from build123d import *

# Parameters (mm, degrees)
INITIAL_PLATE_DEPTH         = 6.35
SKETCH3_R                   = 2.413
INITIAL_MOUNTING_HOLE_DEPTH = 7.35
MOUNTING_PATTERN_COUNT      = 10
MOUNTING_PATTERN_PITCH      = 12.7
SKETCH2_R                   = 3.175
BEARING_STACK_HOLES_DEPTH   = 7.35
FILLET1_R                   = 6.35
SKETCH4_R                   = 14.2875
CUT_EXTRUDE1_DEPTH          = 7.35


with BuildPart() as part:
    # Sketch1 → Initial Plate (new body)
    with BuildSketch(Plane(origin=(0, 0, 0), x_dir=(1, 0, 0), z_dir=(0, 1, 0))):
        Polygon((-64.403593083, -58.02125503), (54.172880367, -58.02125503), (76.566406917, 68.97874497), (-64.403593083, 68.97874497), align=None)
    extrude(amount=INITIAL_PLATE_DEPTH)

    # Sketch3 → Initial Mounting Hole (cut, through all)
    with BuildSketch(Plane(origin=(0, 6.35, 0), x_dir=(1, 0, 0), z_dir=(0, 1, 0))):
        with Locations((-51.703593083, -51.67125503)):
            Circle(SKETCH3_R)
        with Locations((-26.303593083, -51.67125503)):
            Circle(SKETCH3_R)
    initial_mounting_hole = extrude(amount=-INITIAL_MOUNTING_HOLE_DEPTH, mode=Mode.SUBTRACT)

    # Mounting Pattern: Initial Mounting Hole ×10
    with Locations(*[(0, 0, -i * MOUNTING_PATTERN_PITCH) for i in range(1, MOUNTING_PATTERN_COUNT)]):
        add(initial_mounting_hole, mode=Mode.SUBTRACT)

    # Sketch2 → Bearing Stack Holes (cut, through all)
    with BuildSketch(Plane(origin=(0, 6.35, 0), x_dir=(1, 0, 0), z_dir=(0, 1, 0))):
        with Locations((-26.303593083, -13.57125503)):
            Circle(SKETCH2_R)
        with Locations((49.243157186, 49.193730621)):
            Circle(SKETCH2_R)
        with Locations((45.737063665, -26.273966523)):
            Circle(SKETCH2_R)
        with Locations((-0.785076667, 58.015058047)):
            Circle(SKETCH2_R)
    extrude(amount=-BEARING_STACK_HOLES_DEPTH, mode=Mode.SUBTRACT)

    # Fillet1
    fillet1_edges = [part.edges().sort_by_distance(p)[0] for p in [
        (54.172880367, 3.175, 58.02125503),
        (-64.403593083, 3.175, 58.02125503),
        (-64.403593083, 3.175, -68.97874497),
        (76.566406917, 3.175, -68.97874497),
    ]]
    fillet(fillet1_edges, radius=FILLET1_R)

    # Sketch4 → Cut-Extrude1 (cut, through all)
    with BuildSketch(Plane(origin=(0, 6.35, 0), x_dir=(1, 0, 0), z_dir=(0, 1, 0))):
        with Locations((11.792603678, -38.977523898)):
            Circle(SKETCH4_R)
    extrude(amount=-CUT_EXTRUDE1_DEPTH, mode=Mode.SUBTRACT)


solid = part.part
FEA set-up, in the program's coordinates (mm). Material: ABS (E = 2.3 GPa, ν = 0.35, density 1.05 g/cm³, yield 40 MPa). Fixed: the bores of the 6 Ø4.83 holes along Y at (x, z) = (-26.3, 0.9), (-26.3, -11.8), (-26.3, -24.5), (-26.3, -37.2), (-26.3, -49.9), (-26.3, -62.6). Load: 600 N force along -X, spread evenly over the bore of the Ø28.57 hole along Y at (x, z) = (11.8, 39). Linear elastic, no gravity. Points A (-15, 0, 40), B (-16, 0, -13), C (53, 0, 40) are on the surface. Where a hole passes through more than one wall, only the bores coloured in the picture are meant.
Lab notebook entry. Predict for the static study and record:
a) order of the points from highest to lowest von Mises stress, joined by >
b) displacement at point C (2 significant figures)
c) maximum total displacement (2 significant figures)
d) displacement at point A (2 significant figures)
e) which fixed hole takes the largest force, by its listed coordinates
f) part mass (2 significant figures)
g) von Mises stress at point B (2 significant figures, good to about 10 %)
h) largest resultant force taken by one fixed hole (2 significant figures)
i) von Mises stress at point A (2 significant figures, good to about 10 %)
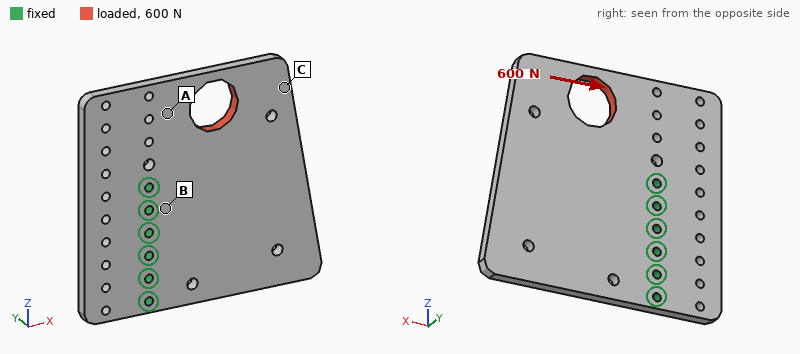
B > A > C
0.23 mm
0.27 mm
0.15 mm
(-26.3, 0.9)
100 g
2.3 MPa
760 N
1.5 MPa
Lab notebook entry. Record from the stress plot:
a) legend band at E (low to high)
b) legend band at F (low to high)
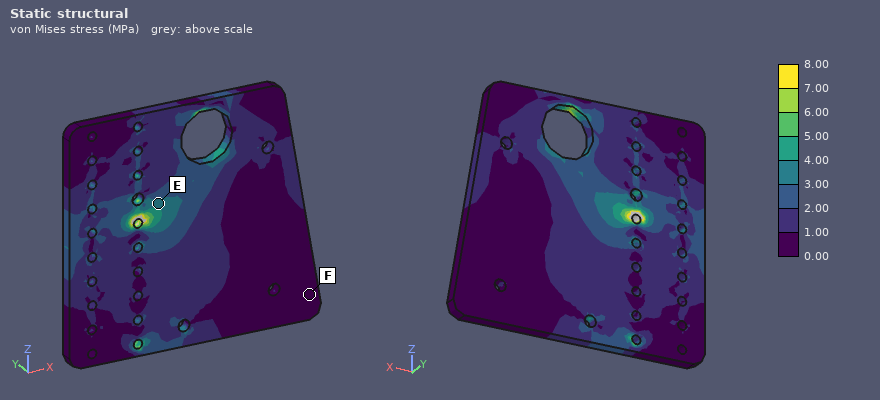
3.00 to 4.00 MPa
0.00 to 1.00 MPa
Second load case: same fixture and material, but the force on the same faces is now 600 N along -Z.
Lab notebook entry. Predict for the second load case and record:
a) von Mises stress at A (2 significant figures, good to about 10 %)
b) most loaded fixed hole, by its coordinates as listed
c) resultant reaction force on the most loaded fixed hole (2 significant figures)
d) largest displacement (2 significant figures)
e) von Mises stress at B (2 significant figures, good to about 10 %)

1.1 MPa
(-26.3, 0.9)
400 N
0.19 mm
2.5 MPa
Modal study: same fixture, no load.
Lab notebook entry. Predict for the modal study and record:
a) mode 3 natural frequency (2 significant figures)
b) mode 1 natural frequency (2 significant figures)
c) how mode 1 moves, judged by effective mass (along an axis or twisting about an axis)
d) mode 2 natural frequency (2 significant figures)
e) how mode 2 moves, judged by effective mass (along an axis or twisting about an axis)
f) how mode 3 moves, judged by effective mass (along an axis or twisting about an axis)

450 Hz
170 Hz
along Y
280 Hz
twisting about X
along Y
